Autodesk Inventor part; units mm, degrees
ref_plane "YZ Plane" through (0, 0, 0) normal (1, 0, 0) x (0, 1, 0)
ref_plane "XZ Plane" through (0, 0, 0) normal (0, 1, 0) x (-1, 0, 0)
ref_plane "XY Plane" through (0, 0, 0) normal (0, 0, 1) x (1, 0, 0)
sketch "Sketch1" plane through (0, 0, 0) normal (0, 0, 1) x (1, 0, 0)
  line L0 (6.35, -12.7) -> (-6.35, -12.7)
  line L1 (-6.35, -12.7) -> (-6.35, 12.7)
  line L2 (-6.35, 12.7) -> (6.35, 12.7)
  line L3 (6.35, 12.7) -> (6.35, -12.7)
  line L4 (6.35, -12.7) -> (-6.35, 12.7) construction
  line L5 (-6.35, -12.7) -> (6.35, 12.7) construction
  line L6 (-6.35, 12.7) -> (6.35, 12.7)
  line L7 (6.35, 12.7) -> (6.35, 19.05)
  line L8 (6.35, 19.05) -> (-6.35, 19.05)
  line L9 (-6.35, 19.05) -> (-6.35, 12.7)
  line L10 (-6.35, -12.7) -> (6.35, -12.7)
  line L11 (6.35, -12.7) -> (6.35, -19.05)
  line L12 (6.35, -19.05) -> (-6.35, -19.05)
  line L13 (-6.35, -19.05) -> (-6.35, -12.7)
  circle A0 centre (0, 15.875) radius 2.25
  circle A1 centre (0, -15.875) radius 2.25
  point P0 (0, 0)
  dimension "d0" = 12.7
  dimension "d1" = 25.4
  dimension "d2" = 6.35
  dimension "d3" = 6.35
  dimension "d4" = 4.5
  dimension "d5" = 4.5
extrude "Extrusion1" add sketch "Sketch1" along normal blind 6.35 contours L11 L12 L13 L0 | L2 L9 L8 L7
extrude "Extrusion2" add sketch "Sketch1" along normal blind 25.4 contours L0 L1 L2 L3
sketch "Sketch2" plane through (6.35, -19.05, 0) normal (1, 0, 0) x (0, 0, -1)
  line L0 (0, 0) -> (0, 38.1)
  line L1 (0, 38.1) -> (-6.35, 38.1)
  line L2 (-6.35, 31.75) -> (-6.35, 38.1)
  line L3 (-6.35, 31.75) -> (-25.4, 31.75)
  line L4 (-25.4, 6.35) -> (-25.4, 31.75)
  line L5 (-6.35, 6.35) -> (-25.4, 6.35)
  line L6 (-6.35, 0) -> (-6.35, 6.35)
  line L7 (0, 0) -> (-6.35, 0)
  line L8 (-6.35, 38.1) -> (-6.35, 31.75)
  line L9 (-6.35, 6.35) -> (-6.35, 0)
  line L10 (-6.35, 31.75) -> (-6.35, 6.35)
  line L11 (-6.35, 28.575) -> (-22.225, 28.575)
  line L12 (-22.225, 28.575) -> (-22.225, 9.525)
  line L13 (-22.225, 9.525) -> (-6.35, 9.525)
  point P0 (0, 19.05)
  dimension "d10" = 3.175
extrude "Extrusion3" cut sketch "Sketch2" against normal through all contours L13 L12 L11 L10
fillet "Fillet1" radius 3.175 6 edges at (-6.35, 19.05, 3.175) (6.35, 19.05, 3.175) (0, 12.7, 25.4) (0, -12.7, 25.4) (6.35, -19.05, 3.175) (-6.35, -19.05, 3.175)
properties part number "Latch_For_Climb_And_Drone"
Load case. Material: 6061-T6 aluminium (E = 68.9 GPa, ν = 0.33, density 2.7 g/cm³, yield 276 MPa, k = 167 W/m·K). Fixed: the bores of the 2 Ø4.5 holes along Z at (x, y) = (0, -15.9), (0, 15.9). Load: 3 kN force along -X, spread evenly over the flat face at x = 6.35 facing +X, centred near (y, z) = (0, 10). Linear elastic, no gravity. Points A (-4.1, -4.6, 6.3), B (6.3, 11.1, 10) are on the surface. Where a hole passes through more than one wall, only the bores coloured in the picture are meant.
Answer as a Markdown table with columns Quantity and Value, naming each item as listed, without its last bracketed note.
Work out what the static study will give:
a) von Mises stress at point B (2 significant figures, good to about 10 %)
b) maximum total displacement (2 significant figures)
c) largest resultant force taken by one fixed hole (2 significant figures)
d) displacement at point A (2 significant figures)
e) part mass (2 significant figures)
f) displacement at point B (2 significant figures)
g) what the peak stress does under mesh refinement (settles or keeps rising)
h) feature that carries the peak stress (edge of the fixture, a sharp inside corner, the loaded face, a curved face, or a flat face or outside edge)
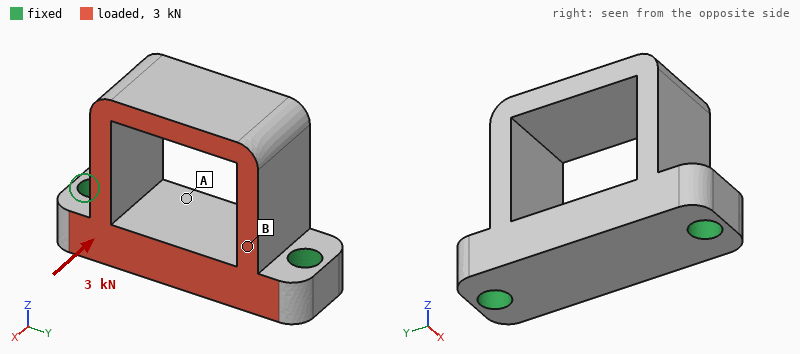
| Quantity | Value |
|---|---|
| von Mises stress at point B | 75 MPa |
| maximum total displacement | 90 µm |
| largest resultant force taken by one fixed hole | 1.5 kN |
| displacement at point A | 16 µm |
| part mass | 14 g |
| displacement at point B | 29 µm |
| what the peak stress does under mesh refinement | keeps rising |
| feature that carries the peak stress | edge of the fixture |
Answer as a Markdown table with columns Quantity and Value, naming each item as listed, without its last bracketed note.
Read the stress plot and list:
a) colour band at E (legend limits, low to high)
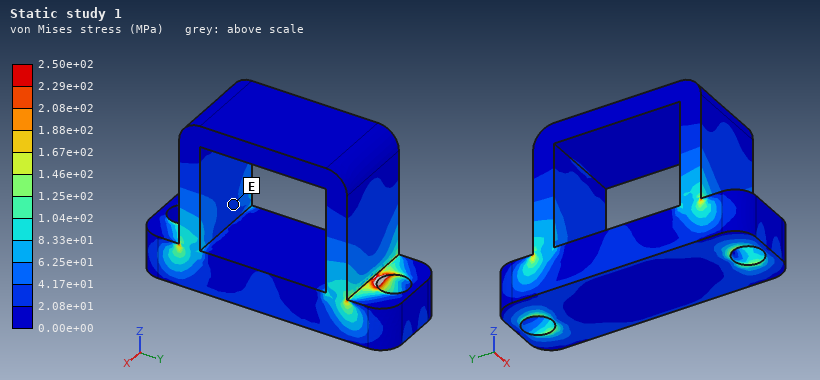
| Quantity | Value |
|---|---|
| colour band at E | 2.08e+01 to 4.17e+01 MPa |
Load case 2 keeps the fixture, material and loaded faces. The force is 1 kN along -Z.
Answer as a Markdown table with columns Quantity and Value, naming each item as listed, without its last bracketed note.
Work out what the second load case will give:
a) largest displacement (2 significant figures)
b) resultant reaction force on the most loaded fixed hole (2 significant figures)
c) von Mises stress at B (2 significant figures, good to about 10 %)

| Quantity | Value |
|---|---|
| largest displacement | 28 µm |
| resultant reaction force on the most loaded fixed hole | 500 N |
| von Mises stress at B | 20 MPa |
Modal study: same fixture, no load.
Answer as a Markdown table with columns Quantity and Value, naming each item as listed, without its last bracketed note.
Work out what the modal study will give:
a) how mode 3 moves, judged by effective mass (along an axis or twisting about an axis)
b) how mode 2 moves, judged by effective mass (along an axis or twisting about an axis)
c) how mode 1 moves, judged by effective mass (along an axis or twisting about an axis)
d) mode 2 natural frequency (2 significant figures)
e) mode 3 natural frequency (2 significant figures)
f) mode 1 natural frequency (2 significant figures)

| Quantity | Value |
|---|---|
| how mode 3 moves, judged by effective mass | twisting about Z |
| how mode 2 moves, judged by effective mass | along X |
| how mode 1 moves, judged by effective mass | along Y |
| mode 2 natural frequency | 9200 Hz |
| mode 3 natural frequency | 14 kHz |
| mode 1 natural frequency | 6600 Hz |
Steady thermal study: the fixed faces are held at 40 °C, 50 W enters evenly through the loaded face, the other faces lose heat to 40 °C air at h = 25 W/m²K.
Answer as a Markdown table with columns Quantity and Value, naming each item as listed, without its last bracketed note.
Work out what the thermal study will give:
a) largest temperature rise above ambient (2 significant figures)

| Quantity | Value |
|---|---|
| largest temperature rise above ambient | 34 K |
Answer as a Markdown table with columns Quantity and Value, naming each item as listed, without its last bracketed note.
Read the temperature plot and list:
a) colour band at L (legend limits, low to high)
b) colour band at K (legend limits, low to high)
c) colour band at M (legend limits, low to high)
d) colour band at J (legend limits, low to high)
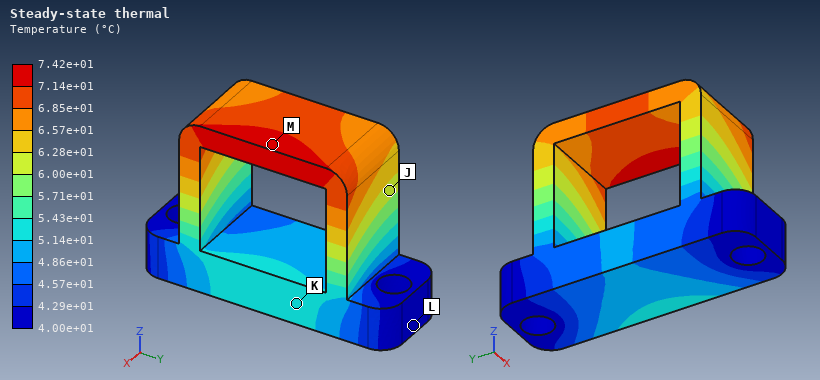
| Quantity | Value |
|---|---|
| colour band at L | 4.00e+01 to 4.29e+01 °C |
| colour band at K | 5.14e+01 to 5.43e+01 °C |
| colour band at M | 7.14e+01 to 7.42e+01 °C |
| colour band at J | 6.00e+01 to 6.28e+01 °C |
